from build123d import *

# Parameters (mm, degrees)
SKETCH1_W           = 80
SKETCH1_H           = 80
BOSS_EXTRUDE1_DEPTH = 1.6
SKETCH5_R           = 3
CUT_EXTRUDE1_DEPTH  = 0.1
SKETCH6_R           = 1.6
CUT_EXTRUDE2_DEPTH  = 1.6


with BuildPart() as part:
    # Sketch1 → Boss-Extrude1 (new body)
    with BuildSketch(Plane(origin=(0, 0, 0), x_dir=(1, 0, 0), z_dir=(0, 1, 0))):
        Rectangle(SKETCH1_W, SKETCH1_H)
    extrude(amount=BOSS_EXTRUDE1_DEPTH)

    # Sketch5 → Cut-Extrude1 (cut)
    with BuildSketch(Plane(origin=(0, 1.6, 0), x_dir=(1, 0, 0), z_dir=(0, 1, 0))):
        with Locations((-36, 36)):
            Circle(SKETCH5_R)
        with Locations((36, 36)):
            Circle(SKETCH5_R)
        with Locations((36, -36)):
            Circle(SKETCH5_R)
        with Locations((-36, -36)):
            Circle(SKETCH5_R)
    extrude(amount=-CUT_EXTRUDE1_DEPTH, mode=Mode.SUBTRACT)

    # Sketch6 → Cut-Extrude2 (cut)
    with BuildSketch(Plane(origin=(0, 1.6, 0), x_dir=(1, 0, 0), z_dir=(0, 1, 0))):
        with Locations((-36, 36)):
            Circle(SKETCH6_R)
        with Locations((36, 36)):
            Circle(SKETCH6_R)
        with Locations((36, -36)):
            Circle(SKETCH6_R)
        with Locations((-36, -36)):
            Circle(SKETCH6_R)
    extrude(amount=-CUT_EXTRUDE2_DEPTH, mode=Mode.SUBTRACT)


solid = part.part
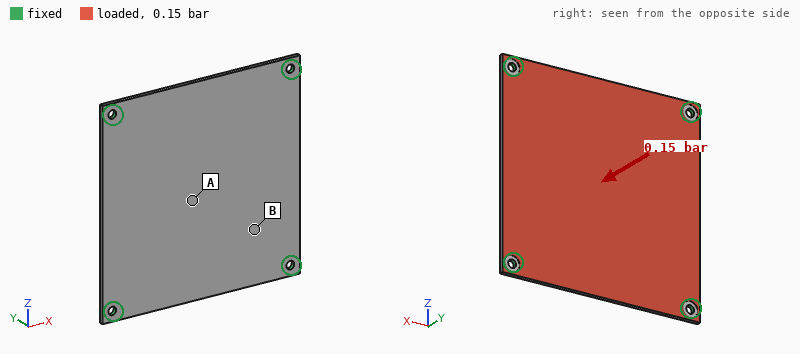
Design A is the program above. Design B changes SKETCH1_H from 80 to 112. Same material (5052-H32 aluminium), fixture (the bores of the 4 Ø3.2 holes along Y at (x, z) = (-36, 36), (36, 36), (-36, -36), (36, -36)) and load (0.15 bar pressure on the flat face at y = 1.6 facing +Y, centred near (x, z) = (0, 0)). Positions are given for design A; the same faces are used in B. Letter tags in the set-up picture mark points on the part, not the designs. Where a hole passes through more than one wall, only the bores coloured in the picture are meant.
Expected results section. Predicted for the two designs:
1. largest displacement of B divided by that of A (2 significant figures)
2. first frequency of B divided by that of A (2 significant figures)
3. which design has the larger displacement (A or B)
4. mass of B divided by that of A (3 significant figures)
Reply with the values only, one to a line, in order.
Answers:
0.89
1.1
A
1.40
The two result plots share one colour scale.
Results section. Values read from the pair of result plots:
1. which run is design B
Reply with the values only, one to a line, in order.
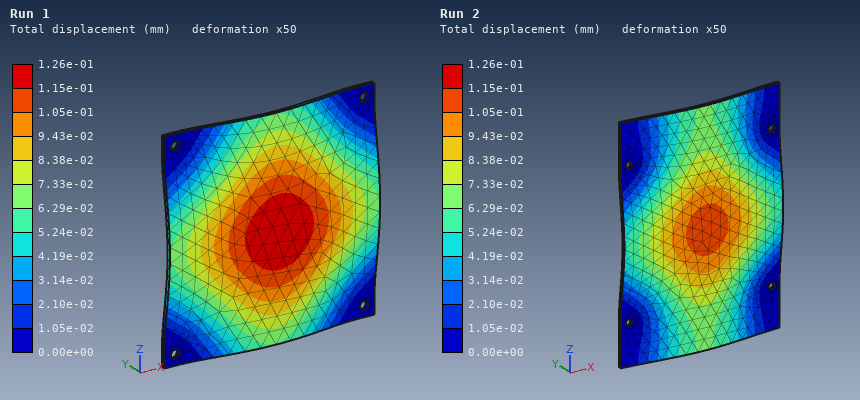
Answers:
Run 2
